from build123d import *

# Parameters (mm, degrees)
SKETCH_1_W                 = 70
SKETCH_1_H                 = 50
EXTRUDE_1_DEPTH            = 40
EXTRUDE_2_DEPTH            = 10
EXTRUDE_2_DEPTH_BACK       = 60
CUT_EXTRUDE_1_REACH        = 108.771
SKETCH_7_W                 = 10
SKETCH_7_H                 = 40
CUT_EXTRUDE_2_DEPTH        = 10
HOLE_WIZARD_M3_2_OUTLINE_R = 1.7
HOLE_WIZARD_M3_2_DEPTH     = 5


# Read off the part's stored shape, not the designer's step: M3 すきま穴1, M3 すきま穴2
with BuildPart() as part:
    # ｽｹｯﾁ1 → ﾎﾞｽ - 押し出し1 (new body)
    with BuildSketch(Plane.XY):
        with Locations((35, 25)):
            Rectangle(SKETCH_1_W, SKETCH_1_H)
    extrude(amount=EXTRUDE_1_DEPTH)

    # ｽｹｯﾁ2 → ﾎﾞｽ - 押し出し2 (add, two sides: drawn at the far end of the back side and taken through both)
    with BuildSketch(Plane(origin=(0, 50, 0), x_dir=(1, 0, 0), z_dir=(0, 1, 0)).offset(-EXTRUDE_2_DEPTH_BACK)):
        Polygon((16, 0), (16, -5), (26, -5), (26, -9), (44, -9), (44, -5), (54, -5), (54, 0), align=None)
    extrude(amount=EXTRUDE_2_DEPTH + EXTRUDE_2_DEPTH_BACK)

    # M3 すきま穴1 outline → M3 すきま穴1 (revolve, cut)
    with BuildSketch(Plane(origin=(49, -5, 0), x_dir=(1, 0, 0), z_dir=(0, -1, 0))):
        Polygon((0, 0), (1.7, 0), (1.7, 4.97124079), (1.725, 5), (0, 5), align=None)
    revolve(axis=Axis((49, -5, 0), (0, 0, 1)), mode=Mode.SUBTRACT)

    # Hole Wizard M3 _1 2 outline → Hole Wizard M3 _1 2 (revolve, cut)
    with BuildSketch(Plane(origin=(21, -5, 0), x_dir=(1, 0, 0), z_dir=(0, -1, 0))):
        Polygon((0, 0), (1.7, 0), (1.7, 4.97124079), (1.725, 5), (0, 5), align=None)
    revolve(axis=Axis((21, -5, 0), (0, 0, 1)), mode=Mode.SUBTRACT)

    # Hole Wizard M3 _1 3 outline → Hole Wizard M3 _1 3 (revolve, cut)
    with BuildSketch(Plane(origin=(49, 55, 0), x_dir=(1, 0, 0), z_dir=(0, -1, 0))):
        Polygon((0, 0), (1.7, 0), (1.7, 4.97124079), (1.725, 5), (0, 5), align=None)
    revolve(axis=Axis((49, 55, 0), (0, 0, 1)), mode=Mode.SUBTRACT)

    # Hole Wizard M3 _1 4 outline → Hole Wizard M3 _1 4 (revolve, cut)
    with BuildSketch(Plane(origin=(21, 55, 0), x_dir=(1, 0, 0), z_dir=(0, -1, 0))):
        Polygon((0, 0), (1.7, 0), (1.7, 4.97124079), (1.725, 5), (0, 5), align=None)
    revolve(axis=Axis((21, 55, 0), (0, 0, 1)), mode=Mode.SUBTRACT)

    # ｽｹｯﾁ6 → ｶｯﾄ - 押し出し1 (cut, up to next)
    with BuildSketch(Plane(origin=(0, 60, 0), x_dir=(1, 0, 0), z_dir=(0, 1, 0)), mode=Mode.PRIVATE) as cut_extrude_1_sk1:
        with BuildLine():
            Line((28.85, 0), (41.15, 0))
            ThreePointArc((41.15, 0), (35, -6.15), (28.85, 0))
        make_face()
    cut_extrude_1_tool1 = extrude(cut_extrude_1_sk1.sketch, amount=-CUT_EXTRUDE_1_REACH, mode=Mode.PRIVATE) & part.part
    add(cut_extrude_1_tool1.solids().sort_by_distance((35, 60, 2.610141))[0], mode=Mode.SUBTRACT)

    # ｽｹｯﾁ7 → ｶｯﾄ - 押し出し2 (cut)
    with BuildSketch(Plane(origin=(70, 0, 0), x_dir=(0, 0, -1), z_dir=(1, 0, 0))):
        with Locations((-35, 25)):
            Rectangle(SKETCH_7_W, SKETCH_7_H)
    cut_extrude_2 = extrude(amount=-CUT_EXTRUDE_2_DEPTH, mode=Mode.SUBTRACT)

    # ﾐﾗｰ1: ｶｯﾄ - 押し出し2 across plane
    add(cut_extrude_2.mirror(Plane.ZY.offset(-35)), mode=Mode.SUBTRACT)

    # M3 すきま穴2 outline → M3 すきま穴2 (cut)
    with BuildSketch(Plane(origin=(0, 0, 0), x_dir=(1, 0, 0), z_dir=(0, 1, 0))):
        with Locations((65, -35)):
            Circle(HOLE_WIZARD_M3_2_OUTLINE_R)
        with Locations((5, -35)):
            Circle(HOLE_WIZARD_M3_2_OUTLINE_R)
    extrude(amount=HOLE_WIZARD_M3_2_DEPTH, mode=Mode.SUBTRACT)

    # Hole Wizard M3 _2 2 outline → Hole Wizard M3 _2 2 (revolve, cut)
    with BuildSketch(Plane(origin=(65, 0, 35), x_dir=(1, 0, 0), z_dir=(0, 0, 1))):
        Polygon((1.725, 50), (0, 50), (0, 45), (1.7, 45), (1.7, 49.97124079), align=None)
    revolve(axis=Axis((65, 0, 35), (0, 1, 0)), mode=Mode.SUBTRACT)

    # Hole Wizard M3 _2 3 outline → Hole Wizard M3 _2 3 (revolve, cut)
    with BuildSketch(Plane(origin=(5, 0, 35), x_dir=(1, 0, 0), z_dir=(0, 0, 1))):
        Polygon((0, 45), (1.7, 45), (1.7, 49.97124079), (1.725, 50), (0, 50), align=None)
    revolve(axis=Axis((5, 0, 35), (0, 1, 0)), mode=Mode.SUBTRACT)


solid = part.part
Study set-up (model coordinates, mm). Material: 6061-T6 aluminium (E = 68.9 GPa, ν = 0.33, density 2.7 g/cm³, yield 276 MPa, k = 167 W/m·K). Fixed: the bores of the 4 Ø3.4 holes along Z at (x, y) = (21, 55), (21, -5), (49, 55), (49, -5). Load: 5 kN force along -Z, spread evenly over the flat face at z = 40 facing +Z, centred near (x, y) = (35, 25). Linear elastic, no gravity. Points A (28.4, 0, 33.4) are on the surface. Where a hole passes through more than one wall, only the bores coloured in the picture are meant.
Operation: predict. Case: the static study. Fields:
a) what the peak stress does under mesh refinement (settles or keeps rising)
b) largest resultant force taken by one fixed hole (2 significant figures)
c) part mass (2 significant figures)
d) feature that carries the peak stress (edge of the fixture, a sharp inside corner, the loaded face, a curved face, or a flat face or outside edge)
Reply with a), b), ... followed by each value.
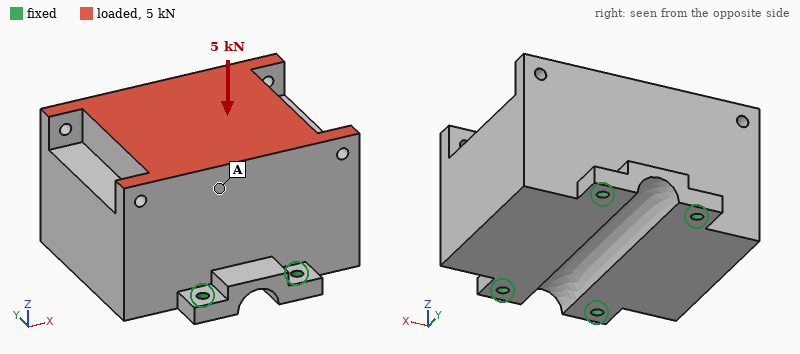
a) keeps rising
b) 1.4 kN
c) 360 g
d) edge of the fixture
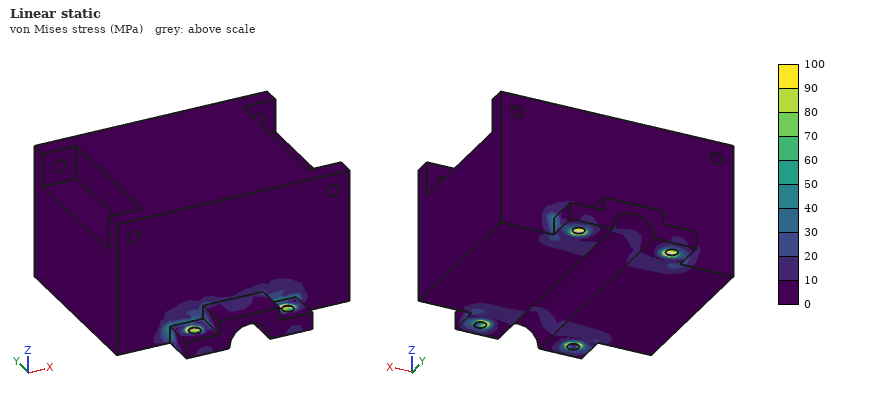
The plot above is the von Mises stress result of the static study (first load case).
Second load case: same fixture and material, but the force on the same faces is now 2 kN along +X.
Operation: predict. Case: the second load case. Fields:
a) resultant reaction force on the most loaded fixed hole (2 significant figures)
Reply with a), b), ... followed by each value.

a) 1.5 kN
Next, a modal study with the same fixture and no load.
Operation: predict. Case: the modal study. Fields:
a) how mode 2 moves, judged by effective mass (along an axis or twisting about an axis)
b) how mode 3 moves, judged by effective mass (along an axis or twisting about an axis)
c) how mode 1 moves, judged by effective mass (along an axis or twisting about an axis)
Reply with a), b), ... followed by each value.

a) along Z
b) along Y
c) along X
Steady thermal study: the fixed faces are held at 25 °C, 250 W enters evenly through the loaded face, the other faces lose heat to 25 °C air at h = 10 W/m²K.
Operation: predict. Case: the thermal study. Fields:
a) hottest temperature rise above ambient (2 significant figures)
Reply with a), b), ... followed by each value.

a) 62 K
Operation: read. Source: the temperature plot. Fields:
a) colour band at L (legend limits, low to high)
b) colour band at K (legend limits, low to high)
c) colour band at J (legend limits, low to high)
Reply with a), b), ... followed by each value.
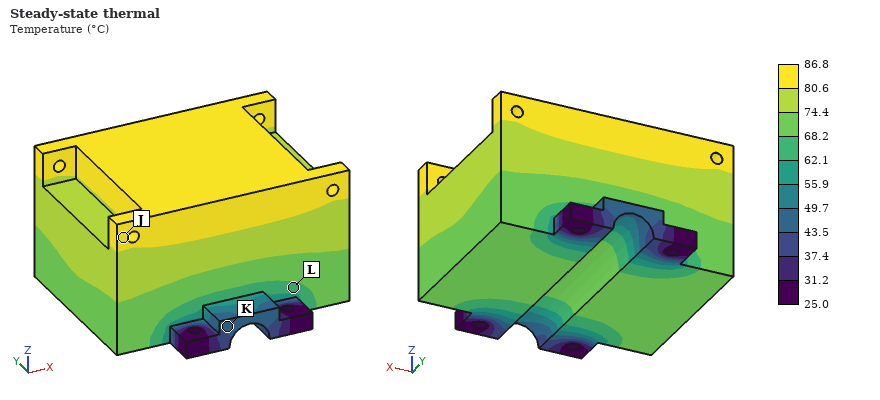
a) 62.1 to 68.2 °C
b) 43.5 to 49.7 °C
c) 80.6 to 86.8 °C
